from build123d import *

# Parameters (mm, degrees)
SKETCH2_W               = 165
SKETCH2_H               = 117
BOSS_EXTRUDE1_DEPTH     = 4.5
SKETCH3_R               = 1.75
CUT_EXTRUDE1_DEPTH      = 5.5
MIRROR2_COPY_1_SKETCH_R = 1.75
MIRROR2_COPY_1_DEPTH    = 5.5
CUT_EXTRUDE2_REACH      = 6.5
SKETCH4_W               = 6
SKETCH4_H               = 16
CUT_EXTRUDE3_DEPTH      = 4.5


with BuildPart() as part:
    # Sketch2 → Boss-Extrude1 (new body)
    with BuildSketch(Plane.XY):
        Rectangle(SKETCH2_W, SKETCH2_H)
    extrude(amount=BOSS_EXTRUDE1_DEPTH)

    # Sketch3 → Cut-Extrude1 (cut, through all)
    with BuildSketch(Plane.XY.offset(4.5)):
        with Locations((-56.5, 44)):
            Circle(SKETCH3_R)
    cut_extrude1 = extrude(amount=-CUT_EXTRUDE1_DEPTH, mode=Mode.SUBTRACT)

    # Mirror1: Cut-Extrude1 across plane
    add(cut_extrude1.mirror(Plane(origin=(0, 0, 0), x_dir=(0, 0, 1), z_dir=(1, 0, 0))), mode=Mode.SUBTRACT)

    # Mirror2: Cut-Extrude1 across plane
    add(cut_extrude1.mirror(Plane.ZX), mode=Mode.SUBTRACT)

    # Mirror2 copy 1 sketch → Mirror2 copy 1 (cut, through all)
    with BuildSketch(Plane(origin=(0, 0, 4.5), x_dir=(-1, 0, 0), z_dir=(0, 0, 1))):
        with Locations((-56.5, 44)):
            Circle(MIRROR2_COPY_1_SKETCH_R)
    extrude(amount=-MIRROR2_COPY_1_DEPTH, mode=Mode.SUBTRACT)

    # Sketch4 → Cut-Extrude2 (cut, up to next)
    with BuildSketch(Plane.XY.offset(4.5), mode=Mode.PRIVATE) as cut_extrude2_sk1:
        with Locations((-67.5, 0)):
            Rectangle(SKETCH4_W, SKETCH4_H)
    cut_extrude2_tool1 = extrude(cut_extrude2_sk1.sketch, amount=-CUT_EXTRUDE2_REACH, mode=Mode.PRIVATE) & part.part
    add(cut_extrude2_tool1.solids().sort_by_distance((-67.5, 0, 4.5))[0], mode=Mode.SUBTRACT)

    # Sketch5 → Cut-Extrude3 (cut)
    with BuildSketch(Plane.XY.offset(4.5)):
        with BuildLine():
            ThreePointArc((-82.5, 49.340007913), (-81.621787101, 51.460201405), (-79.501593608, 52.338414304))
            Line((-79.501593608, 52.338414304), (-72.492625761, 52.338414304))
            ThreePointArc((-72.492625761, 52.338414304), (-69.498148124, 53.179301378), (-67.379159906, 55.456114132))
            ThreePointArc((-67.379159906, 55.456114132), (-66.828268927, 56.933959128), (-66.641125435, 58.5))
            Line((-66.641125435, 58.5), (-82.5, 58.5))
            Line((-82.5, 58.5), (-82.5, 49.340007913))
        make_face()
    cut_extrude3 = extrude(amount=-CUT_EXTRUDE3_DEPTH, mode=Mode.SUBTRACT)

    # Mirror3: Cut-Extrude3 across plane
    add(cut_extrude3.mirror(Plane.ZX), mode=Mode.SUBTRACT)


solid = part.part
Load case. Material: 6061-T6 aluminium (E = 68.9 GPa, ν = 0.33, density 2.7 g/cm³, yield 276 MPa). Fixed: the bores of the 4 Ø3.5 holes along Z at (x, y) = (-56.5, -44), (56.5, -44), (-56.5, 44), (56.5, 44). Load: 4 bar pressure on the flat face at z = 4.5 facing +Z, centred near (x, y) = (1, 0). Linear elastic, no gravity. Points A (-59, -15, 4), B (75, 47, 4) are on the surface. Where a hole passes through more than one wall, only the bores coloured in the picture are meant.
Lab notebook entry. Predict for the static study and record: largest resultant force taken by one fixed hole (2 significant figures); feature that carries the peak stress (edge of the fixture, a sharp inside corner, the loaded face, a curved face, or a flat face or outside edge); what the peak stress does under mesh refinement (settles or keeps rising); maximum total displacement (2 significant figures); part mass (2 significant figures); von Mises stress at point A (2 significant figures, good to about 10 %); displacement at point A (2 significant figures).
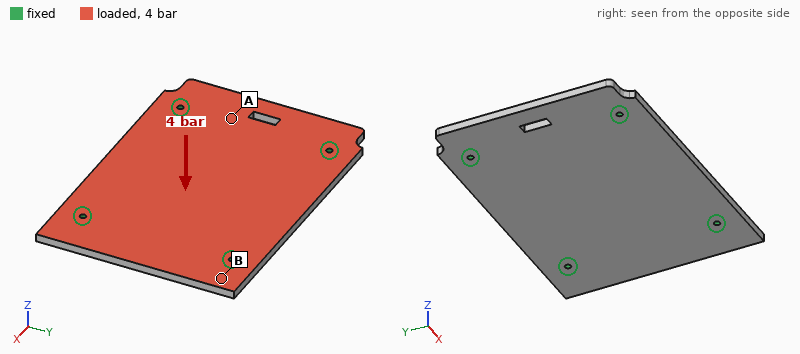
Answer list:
1.9 kN
edge of the fixture
keeps rising
0.59 mm
230 g
51 MPa
0.18 mm
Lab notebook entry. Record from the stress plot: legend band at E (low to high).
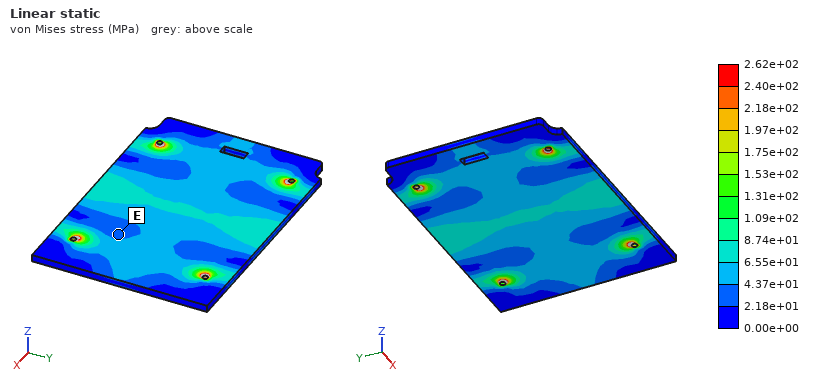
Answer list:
2.18e+01 to 4.37e+01 MPa
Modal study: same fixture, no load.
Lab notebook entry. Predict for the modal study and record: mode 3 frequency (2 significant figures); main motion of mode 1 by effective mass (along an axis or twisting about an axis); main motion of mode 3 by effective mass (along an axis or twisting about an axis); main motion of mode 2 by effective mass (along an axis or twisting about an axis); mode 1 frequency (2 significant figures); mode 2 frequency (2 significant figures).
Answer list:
2300 Hz
along Z
along Z
twisting about X
1400 Hz
2000 Hz
